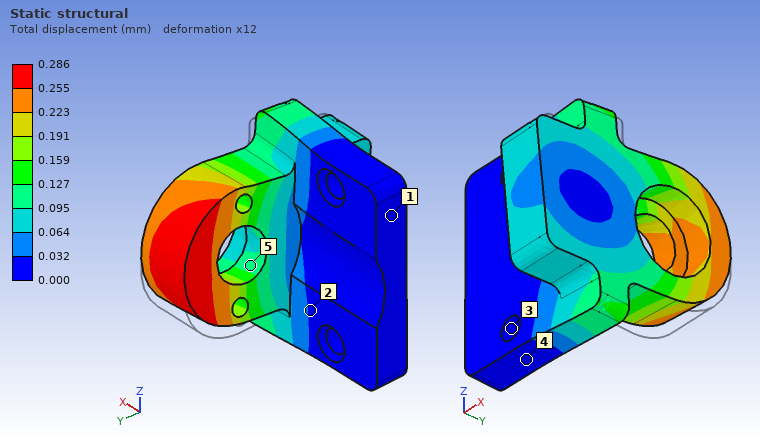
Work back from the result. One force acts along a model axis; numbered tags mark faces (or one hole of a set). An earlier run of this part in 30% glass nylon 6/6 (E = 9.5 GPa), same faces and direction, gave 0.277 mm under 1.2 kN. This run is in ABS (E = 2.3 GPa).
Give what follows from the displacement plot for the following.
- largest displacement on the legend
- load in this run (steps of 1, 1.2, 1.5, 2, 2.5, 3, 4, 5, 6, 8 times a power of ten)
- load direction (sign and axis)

0.286 mm
300 N
+Z
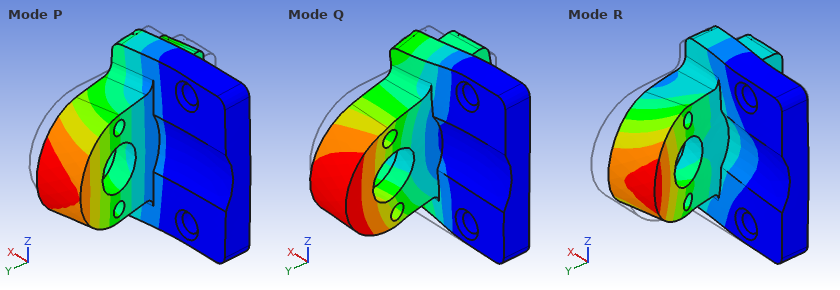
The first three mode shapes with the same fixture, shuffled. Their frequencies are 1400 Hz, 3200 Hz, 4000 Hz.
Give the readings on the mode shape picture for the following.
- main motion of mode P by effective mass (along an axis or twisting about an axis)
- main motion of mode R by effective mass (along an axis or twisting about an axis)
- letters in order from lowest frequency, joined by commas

along Y
along Y
P, Q, R
